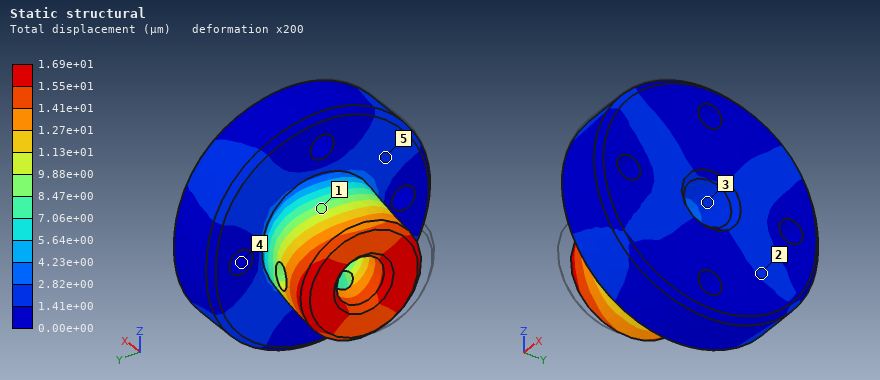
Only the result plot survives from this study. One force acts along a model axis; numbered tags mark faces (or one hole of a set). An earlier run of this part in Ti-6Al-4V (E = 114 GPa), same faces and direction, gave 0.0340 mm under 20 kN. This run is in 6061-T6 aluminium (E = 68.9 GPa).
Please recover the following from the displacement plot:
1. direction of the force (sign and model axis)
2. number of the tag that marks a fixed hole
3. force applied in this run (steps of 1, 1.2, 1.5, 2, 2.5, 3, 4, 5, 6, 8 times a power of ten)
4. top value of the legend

+Y
4
6 kN
1.69e+01 µm
